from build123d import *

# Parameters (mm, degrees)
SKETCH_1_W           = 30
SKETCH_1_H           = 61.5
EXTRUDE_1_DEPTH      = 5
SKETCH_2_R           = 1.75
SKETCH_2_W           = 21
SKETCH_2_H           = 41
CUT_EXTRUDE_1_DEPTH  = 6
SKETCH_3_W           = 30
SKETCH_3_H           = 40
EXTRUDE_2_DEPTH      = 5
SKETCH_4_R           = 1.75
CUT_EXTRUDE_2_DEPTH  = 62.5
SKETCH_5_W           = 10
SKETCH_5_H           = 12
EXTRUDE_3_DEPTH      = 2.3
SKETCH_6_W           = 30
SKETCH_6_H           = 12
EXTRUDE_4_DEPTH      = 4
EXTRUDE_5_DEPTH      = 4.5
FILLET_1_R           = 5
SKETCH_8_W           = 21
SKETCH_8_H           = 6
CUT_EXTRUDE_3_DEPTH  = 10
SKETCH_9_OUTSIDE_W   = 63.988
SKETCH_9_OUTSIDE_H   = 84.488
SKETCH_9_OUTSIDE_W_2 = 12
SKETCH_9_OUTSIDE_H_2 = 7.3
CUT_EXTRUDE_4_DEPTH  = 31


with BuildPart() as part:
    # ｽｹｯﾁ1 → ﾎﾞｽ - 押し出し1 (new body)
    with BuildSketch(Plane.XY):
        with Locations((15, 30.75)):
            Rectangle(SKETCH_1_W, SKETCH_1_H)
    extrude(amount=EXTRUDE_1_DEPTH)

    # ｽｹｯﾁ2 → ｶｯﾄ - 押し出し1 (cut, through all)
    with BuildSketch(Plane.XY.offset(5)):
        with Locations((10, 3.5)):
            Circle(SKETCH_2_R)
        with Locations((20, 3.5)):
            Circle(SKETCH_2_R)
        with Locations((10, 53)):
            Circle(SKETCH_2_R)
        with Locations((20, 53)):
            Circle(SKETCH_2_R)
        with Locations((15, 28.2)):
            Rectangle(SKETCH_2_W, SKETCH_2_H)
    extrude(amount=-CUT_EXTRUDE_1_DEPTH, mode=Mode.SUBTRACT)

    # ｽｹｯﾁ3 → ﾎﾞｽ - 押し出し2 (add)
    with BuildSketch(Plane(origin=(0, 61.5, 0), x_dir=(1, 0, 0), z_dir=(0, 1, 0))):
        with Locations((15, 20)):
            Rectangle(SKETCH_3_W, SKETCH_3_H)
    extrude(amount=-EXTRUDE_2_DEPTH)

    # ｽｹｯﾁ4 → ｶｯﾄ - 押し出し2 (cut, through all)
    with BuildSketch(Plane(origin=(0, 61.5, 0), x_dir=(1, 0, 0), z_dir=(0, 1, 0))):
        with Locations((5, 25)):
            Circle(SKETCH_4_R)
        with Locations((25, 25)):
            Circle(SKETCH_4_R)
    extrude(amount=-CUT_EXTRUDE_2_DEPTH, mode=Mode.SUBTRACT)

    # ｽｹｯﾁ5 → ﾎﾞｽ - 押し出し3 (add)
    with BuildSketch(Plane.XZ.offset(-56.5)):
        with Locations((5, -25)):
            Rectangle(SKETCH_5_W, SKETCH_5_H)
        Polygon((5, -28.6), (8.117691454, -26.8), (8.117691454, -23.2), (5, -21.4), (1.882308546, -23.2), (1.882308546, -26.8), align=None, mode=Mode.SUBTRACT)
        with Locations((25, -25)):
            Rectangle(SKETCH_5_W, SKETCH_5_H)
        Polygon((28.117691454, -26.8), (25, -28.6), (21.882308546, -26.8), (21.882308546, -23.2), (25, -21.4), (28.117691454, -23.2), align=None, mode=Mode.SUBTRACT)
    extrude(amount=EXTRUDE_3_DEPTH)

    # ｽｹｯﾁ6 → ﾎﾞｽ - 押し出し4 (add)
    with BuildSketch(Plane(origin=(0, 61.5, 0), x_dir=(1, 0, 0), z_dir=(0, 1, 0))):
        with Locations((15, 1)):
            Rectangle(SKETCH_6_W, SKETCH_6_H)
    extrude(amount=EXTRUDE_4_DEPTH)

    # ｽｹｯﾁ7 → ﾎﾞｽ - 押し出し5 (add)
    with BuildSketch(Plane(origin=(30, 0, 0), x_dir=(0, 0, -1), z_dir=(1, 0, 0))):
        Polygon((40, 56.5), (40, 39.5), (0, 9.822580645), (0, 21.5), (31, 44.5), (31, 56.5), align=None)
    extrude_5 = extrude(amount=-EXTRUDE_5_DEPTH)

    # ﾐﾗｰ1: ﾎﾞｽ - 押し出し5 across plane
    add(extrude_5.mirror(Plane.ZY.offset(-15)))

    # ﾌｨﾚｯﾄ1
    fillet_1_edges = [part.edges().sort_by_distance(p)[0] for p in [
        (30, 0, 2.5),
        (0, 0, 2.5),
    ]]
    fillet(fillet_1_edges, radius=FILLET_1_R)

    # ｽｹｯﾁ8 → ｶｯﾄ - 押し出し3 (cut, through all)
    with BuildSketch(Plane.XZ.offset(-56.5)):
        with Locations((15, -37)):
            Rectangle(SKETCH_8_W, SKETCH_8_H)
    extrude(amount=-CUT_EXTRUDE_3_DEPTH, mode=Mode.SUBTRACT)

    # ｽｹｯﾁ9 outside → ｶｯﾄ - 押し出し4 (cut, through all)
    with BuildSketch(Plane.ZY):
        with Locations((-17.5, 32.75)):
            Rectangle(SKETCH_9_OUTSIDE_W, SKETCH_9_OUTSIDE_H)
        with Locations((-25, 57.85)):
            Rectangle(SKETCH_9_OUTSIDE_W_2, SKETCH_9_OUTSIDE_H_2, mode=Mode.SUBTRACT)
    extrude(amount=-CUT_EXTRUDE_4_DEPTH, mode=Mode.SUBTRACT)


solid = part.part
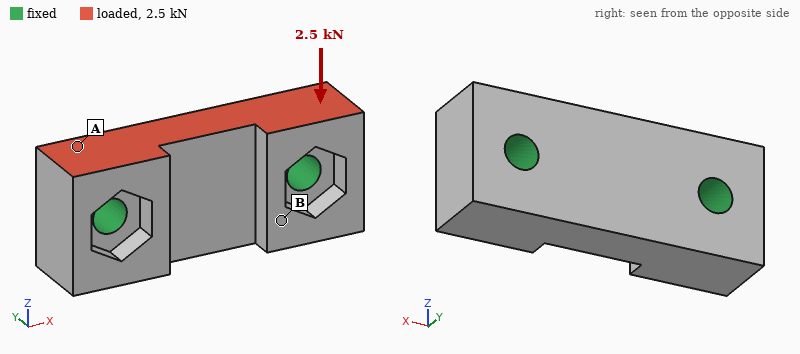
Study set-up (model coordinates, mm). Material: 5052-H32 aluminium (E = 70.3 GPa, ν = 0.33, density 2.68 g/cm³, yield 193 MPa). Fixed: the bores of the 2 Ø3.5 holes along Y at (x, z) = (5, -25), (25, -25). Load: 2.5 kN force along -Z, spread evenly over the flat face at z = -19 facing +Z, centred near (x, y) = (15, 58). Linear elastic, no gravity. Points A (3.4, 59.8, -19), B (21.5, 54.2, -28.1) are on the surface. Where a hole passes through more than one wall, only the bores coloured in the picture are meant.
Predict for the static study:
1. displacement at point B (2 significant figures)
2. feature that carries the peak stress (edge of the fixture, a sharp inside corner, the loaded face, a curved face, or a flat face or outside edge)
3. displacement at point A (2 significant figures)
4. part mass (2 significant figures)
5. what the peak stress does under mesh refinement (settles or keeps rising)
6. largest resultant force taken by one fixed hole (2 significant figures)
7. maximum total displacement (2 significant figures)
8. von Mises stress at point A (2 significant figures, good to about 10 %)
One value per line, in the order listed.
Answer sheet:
2.2 µm
edge of the fixture
1.6 µm
5.6 g
keeps rising
1.3 kN
4.3 µm
19 MPa
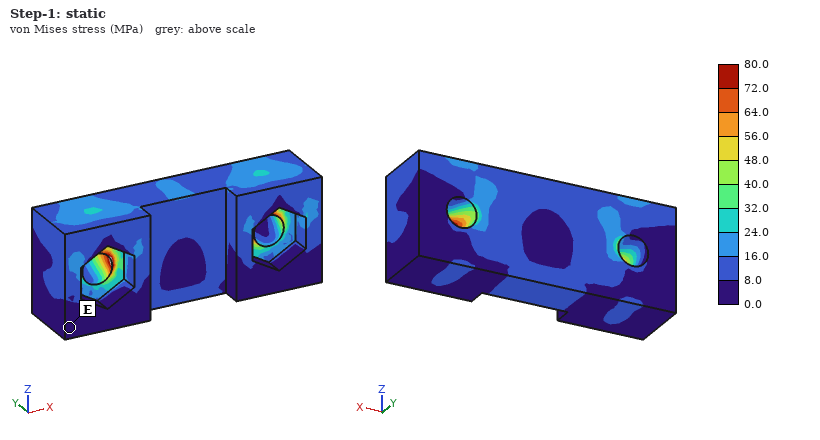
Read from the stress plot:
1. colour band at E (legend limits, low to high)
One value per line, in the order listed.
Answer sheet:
0.0 to 8.0 MPa
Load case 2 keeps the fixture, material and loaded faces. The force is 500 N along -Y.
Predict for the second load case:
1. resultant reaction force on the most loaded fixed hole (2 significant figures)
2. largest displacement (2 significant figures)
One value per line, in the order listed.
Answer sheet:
250 N
4.3 µm
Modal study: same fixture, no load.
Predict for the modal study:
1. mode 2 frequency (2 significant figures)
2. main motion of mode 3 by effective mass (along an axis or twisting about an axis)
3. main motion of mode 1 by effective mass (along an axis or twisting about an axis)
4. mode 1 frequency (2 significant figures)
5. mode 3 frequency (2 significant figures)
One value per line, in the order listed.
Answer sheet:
52 kHz
along Z
along Y
48 kHz
58 kHz
